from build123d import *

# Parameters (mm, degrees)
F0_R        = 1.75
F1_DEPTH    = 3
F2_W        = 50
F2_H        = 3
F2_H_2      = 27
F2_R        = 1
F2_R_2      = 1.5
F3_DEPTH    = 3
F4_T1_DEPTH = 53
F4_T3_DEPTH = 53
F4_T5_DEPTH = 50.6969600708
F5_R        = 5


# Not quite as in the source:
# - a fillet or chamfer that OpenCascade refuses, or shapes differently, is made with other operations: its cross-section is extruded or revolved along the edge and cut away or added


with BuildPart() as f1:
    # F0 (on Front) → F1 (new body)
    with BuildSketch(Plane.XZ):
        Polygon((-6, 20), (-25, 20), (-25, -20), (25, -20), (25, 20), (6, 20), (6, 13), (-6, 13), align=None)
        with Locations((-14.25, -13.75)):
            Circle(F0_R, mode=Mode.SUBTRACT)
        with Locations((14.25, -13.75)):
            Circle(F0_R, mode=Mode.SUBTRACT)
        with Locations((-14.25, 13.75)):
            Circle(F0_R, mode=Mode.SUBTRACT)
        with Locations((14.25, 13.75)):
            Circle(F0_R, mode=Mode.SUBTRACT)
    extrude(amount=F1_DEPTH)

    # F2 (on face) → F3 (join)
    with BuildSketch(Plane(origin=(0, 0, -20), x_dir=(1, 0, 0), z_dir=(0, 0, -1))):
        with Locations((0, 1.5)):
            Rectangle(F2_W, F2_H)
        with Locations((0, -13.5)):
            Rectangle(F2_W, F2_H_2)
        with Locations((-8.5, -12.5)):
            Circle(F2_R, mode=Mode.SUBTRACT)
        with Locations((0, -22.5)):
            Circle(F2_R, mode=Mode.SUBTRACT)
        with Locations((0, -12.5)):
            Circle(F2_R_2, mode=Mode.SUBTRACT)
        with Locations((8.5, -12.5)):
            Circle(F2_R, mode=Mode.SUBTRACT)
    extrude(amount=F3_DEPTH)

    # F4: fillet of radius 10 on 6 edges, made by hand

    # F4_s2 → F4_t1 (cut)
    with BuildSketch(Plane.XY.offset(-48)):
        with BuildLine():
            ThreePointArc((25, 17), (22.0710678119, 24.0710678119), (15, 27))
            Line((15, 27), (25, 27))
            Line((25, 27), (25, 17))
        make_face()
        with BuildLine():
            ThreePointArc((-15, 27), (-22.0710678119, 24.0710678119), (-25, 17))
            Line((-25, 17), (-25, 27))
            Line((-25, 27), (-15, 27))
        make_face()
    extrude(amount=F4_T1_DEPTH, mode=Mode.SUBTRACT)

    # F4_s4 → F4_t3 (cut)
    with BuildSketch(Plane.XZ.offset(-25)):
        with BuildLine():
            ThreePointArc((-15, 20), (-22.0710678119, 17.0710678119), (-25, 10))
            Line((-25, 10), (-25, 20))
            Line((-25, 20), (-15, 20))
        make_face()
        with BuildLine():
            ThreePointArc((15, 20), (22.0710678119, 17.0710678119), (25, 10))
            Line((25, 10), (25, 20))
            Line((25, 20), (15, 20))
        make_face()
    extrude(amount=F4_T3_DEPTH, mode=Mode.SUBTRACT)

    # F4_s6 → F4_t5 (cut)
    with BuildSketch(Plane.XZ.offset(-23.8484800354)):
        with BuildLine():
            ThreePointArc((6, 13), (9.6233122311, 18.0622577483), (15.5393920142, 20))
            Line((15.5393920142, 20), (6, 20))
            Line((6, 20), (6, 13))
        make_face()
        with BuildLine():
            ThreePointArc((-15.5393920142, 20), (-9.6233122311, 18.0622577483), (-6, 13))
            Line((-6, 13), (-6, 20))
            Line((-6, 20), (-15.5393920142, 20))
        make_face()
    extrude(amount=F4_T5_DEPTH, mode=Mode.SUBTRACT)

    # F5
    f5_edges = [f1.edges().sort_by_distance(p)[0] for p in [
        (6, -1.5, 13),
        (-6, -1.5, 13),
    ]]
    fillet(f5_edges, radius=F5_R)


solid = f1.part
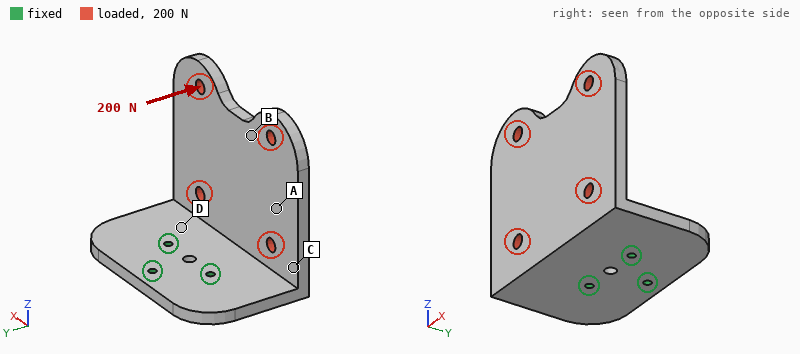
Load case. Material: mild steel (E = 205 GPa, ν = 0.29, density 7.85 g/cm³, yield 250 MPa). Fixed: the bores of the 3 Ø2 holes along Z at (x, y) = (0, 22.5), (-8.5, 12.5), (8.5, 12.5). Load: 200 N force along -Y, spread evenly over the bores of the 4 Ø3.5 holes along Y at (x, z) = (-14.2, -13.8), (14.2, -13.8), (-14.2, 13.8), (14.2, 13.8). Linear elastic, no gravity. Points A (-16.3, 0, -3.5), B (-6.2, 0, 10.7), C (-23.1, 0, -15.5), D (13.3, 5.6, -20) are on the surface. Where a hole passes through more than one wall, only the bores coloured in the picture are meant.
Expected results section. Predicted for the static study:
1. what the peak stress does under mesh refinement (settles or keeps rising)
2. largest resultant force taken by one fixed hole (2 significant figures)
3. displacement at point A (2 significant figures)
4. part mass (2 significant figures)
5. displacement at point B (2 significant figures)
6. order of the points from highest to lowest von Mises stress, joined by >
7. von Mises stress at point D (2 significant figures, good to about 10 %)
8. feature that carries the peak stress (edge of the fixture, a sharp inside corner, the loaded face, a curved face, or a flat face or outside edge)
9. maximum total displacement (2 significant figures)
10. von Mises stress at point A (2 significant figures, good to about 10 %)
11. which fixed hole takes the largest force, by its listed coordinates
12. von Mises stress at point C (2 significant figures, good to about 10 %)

keeps rising
130 N
0.075 mm
76 g
0.15 mm
D > C > A > B
54 MPa
edge of the fixture
0.20 mm
22 MPa
(0, 22.5)
40 MPa
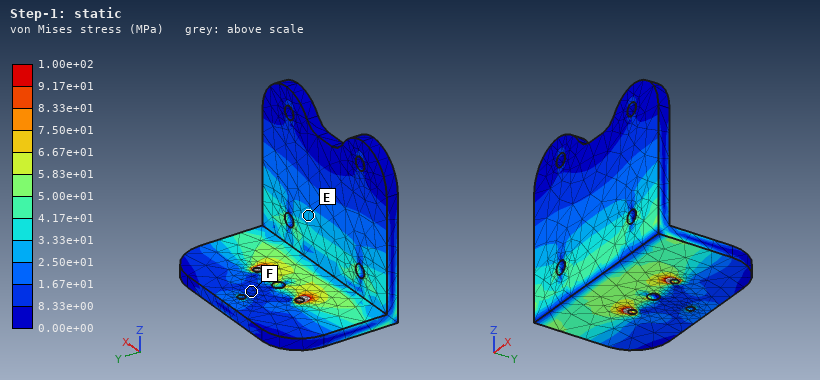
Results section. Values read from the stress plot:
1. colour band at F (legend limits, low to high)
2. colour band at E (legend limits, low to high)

8.33e+00 to 1.67e+01 MPa
2.50e+01 to 3.33e+01 MPa
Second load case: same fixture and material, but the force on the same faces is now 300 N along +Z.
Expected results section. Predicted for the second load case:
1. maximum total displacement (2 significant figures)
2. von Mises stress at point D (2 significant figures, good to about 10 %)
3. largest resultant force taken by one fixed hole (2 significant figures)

74 µm
27 MPa
210 N
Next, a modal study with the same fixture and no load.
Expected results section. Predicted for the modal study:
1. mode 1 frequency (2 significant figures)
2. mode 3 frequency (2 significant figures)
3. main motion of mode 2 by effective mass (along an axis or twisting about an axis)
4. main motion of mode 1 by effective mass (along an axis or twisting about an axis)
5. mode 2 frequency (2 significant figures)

1000 Hz
3000 Hz
along X
along Y
1900 Hz
